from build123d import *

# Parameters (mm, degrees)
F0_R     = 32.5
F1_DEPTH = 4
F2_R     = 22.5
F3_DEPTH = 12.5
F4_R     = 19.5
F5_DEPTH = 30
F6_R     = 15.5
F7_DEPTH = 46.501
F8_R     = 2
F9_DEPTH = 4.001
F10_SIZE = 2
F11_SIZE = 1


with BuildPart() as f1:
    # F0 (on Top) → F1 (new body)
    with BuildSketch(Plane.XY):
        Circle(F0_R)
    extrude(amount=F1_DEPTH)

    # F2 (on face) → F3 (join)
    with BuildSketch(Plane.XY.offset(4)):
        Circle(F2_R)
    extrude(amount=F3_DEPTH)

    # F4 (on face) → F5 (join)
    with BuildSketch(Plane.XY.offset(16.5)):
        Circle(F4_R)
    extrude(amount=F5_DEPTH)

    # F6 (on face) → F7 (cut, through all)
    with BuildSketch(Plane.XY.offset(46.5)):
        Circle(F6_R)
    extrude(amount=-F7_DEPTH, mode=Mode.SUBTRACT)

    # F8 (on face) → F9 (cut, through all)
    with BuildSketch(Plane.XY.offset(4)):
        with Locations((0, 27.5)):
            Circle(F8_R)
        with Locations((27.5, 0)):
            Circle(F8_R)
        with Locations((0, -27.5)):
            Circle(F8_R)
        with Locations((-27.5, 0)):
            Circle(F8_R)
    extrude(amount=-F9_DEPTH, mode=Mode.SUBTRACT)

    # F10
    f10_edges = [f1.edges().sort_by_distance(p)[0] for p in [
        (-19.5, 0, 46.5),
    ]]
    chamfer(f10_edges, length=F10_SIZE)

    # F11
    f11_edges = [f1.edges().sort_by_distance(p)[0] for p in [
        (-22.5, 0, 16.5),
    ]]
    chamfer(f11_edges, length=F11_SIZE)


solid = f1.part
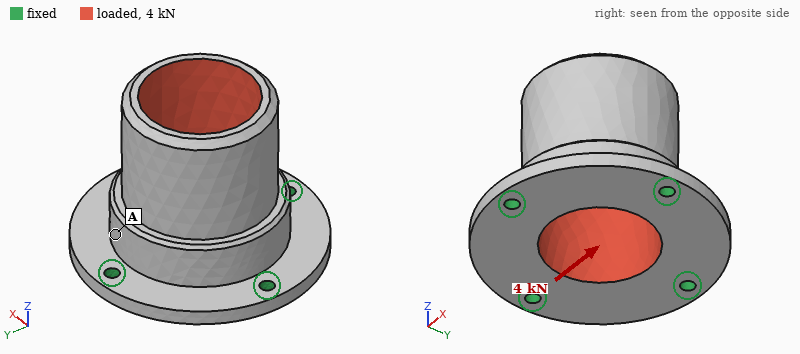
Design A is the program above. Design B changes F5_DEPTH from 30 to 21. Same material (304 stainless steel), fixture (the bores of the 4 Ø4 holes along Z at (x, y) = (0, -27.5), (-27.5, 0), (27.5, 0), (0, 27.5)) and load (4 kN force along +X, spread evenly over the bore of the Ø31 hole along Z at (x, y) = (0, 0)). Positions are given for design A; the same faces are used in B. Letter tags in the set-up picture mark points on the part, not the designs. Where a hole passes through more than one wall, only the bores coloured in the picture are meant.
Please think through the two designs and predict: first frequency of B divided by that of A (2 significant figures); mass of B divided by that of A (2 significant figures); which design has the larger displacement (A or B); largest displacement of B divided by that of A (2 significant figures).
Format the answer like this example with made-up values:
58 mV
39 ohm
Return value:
1.3
0.88
A
0.66
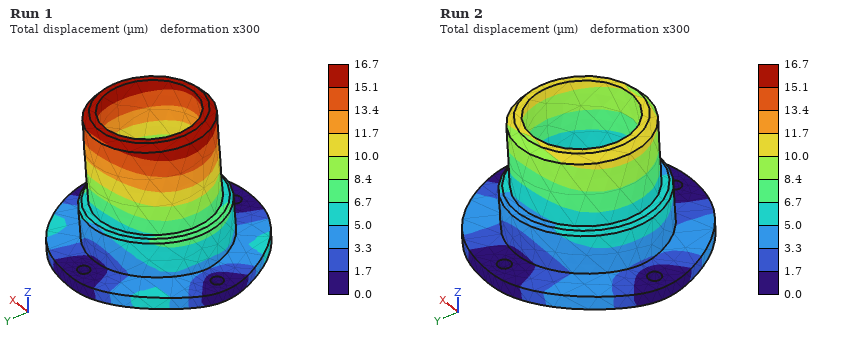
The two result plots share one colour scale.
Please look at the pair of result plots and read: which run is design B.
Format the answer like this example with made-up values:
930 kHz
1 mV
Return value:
Run 2
